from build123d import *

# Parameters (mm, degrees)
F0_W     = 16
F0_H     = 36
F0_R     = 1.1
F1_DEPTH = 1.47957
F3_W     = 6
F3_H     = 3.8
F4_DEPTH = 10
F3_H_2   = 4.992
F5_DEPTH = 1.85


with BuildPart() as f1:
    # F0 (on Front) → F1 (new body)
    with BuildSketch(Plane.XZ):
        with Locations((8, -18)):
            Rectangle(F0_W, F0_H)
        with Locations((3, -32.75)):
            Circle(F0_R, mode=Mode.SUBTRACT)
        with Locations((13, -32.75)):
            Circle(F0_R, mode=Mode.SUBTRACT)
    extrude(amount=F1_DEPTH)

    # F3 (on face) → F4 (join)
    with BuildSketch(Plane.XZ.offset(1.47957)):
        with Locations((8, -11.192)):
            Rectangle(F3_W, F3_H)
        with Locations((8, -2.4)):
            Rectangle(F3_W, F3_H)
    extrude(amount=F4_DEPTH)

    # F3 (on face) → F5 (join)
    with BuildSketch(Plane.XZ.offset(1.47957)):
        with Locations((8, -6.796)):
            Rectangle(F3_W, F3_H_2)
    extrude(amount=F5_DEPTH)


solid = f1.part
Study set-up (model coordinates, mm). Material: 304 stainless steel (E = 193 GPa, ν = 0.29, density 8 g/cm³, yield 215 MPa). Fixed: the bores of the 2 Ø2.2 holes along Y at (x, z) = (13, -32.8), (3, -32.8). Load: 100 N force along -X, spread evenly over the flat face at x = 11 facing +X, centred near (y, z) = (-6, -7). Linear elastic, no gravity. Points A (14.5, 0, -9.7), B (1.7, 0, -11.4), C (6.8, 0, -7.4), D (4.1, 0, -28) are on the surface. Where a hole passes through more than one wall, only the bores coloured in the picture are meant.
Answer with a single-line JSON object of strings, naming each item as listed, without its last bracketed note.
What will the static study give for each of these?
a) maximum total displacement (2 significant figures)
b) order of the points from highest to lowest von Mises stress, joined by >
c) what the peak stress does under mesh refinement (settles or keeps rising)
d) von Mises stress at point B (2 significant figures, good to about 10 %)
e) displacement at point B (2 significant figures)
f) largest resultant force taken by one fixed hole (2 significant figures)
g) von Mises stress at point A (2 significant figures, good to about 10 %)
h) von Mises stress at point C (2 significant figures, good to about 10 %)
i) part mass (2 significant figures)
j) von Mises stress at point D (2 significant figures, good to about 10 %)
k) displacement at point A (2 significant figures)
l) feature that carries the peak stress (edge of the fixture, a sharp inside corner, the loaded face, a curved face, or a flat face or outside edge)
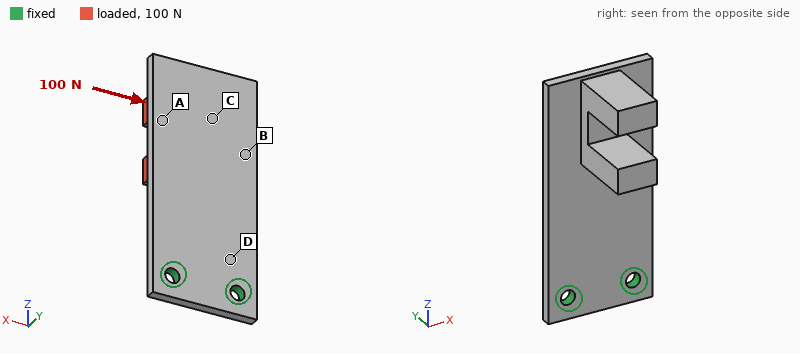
{"maximum total displacement": "87 µm", "order of the points from highest to lowest von Mises stress, joined by >": "D > B > A > C", "what the peak stress does under mesh refinement": "keeps rising", "von Mises stress at point B": "45 MPa", "displacement at point B": "39 µm", "largest resultant force taken by one fixed hole": "240 N", "von Mises stress at point A": "34 MPa", "von Mises stress at point C": "16 MPa", "part mass": "11 g", "von Mises stress at point D": "59 MPa", "displacement at point A": "42 µm", "feature that carries the peak stress": "edge of the fixture"}
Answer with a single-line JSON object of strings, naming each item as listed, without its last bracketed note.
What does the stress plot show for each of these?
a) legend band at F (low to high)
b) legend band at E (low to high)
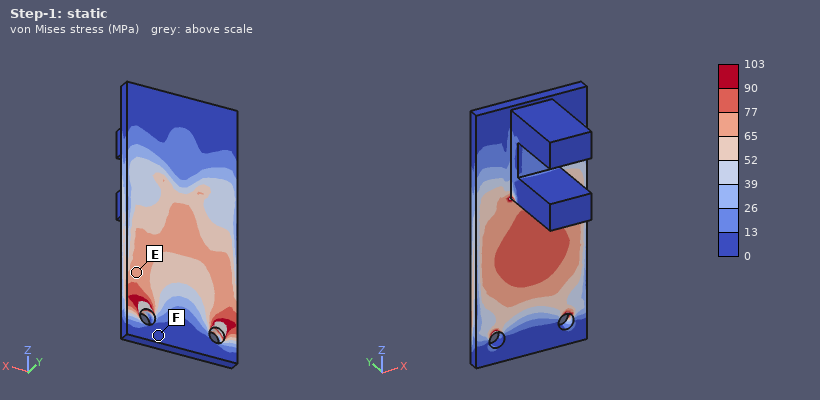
{"legend band at F": "0 to 13 MPa", "legend band at E": "65 to 77 MPa"}
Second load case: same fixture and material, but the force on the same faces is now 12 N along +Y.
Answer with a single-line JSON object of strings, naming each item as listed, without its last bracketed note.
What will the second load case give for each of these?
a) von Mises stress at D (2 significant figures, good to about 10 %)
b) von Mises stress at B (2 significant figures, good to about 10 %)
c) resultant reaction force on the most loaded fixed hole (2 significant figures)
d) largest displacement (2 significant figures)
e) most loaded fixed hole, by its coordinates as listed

{"von Mises stress at D": "39 MPa", "von Mises stress at B": "8.2 MPa", "resultant reaction force on the most loaded fixed hole": "9.1 N", "largest displacement": "0.12 mm", "most loaded fixed hole, by its coordinates as listed": "(13, -32.8)"}
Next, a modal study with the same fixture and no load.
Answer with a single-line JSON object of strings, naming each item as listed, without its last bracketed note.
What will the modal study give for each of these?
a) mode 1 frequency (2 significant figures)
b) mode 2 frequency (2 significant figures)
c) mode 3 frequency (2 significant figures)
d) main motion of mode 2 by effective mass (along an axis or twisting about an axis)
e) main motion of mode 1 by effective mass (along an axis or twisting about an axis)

{"mode 1 frequency": "700 Hz", "mode 2 frequency": "2800 Hz", "mode 3 frequency": "4700 Hz", "main motion of mode 2 by effective mass": "along X", "main motion of mode 1 by effective mass": "along Y"}
